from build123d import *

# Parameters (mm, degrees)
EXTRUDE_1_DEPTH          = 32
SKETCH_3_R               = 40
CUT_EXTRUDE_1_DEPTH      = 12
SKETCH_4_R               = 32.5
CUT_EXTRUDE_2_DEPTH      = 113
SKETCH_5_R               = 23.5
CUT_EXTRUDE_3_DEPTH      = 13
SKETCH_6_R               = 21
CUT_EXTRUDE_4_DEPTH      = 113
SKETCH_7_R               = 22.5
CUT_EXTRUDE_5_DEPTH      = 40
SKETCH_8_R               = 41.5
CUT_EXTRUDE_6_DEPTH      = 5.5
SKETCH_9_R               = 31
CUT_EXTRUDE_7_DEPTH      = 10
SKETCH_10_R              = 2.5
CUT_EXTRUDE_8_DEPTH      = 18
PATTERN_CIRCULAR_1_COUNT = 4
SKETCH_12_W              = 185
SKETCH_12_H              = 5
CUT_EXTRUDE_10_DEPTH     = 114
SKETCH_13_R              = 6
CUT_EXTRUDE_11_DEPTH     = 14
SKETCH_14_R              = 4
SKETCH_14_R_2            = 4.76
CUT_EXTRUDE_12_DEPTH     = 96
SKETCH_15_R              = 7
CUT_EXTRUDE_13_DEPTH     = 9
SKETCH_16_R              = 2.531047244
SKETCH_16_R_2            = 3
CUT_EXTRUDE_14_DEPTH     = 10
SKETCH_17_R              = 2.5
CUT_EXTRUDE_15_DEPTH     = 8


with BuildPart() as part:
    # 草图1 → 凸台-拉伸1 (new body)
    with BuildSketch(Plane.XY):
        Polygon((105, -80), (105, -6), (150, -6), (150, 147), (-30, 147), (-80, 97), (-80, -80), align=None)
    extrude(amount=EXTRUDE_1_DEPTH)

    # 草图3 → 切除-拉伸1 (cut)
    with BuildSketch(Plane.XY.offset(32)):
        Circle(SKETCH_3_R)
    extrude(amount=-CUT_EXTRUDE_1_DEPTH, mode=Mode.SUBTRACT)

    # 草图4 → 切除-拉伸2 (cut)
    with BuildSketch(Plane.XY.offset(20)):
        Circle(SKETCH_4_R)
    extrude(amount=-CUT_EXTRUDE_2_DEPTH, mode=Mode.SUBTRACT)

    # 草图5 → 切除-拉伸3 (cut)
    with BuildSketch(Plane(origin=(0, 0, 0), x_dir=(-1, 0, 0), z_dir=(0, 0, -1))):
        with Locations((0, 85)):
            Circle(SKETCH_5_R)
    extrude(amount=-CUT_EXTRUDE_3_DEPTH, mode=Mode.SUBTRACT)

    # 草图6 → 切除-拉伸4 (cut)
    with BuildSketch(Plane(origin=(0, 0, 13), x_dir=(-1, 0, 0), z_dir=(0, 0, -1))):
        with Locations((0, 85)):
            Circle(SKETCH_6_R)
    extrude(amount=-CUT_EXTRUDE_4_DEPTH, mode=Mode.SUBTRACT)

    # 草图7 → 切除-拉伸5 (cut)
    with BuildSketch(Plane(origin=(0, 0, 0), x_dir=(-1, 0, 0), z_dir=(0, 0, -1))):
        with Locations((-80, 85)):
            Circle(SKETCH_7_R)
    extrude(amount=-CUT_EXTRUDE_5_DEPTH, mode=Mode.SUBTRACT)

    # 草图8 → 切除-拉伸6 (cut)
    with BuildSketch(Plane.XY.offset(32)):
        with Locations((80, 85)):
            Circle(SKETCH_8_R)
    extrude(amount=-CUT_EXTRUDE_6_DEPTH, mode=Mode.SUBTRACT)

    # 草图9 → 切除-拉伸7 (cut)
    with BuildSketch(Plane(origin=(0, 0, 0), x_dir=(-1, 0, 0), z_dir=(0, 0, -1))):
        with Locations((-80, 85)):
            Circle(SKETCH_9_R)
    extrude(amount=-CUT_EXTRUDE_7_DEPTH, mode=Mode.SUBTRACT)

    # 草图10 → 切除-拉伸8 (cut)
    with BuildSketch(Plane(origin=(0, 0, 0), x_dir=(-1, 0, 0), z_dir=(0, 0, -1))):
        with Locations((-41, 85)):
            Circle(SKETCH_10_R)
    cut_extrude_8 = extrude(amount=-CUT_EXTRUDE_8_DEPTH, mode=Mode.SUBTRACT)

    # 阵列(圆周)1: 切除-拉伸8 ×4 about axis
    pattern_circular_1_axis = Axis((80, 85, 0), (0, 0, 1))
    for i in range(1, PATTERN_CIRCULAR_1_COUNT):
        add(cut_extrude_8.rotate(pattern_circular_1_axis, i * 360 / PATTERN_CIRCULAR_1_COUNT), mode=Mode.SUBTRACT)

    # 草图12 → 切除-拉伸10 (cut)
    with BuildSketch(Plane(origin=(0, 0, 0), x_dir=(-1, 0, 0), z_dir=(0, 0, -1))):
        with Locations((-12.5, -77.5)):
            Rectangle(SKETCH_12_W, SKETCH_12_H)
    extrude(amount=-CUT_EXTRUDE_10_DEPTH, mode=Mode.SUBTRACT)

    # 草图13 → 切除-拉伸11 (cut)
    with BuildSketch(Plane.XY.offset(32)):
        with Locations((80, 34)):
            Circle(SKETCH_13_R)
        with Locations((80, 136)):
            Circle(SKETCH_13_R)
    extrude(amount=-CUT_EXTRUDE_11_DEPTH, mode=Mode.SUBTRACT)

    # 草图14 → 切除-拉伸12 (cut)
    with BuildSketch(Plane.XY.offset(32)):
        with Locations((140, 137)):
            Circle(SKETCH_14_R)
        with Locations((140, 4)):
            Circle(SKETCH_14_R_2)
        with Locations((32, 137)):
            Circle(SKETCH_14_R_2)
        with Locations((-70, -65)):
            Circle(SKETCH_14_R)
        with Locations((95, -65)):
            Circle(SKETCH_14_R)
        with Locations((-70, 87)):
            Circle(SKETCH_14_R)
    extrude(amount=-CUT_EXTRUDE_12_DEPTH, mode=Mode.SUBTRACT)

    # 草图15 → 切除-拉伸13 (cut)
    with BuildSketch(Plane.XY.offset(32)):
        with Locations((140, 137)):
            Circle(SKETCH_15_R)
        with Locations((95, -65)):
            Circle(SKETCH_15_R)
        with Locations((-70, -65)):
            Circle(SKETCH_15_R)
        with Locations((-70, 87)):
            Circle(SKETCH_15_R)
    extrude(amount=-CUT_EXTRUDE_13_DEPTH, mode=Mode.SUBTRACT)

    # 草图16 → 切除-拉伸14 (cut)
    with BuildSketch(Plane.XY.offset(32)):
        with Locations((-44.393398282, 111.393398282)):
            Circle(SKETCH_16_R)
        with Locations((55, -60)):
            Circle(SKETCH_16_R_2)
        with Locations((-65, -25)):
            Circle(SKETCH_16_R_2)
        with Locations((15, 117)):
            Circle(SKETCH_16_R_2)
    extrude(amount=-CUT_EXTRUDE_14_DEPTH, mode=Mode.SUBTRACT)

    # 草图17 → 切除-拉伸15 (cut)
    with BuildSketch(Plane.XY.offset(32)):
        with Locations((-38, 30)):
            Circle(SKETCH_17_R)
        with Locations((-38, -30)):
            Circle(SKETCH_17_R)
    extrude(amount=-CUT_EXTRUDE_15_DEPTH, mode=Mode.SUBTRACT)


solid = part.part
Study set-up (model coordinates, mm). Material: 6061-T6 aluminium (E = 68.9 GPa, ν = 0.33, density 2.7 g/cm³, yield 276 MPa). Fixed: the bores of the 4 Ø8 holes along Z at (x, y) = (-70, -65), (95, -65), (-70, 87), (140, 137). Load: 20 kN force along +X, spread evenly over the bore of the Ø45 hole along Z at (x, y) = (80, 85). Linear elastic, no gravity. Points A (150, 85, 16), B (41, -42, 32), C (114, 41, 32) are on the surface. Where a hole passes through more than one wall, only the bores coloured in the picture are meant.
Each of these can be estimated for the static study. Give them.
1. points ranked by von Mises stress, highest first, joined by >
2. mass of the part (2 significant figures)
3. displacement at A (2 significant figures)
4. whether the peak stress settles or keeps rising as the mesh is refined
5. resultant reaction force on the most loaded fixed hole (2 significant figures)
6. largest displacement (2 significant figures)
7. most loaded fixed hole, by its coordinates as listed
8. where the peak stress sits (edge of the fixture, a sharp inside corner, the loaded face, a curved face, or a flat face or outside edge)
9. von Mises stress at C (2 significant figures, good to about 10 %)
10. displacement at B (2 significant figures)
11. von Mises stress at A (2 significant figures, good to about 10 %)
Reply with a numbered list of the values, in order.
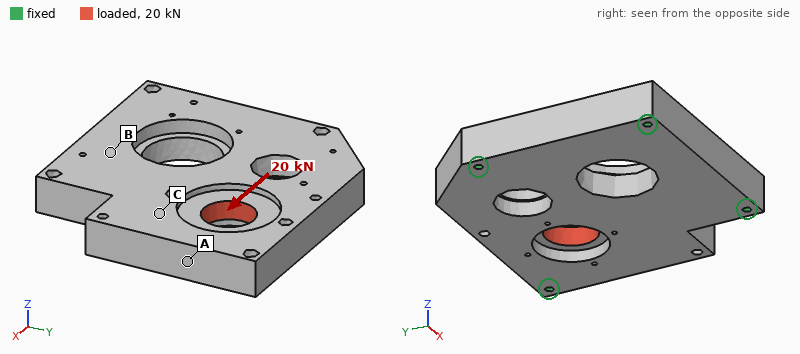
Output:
1. A > C > B
2. 3.3 kg
3. 13 µm
4. keeps rising
5. 8.7 kN
6. 18 µm
7. (140, 137)
8. edge of the fixture
9. 3.5 MPa
10. 3.3 µm
11. 8.1 MPa
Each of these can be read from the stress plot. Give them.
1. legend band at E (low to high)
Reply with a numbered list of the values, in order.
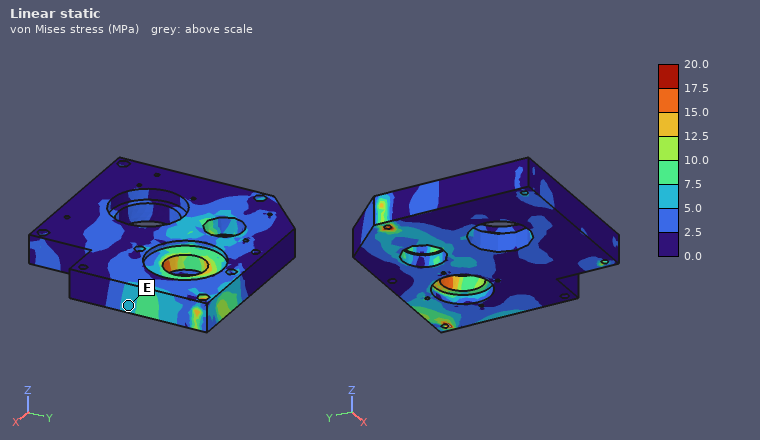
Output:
1. 5.0 to 7.5 MPa
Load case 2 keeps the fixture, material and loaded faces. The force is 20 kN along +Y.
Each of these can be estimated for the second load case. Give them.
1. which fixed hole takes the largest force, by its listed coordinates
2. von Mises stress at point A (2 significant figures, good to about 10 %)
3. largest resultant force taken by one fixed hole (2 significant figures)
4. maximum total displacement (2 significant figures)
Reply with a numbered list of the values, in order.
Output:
1. (140, 137)
2. 7.3 MPa
3. 9.0 kN
4. 21 µm
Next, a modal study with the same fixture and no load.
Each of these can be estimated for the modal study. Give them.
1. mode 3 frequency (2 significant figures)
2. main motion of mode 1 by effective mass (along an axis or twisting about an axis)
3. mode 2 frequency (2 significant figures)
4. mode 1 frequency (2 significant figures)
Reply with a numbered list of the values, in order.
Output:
1. 3200 Hz
2. along Z
3. 2500 Hz
4. 2000 Hz
